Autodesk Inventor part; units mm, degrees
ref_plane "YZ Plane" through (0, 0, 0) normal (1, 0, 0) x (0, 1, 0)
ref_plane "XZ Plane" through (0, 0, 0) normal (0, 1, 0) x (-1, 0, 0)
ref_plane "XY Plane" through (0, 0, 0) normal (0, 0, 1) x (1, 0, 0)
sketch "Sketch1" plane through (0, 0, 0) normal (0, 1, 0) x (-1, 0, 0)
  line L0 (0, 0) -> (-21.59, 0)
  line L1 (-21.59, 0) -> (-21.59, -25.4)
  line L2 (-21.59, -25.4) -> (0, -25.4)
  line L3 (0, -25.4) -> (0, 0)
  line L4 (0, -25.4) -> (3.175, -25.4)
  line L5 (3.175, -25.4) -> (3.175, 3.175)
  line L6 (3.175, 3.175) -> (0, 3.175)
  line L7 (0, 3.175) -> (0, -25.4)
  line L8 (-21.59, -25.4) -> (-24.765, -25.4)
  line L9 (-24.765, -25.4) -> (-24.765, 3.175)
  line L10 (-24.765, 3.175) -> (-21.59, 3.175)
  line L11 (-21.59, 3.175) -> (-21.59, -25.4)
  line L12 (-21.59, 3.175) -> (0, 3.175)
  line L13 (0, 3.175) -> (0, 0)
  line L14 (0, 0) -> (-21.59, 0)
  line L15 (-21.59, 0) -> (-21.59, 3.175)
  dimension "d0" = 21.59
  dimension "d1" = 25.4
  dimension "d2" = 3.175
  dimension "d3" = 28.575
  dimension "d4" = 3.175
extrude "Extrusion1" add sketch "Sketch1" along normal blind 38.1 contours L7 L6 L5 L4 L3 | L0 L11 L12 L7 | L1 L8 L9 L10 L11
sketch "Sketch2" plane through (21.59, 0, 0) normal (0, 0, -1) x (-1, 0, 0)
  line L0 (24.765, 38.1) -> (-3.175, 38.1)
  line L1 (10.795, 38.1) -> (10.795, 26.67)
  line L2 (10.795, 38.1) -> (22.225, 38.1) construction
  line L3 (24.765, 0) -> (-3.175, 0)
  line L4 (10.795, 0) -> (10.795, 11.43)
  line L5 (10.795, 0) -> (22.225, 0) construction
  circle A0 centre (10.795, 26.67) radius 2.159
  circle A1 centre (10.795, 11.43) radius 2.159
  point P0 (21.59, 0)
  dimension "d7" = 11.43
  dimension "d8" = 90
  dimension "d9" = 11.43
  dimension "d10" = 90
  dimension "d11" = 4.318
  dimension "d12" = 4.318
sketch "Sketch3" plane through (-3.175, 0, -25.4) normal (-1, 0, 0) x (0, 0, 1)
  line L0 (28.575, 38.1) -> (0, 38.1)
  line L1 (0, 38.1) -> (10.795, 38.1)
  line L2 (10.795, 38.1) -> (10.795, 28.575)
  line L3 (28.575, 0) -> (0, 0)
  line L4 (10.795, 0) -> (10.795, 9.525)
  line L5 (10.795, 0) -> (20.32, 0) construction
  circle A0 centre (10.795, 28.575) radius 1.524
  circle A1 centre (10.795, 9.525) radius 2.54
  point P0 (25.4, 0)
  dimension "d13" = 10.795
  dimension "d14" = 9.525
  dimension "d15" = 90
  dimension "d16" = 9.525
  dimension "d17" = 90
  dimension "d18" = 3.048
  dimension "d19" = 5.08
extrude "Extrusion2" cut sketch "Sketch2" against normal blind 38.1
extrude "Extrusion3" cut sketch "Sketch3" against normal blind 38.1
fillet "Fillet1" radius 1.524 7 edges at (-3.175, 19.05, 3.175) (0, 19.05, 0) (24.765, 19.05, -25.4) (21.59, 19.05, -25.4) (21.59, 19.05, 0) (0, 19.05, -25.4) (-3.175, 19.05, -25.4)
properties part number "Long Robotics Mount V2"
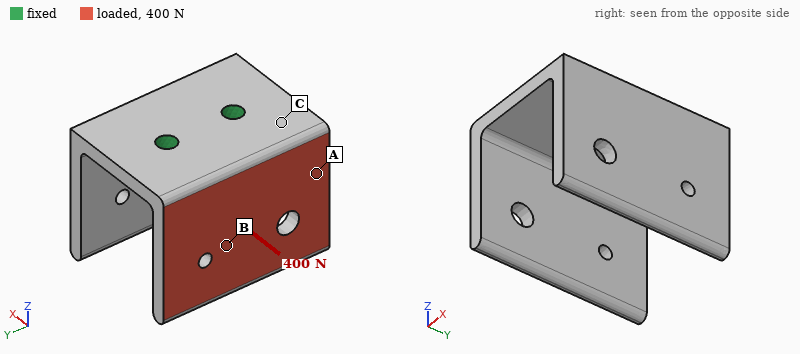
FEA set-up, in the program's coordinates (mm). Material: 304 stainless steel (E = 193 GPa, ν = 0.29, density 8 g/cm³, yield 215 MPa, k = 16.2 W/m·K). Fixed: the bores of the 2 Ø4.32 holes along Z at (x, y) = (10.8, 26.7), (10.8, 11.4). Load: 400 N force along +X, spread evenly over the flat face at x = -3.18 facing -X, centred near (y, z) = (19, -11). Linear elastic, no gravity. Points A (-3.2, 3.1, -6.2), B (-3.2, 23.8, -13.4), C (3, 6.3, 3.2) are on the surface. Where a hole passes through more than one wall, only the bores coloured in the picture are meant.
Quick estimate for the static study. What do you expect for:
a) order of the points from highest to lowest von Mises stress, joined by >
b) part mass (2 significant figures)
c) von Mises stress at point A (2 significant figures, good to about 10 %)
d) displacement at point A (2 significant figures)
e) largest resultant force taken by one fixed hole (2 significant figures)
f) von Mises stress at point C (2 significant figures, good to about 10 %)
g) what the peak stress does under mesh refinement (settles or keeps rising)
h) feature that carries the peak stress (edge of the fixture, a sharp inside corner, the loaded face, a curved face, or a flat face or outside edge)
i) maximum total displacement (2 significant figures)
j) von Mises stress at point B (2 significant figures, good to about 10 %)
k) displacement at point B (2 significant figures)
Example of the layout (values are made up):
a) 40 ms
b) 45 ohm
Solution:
a) C > A > B
b) 74 g
c) 37 MPa
d) 0.034 mm
e) 200 N
f) 65 MPa
g) keeps rising
h) edge of the fixture
i) 0.11 mm
j) 14 MPa
k) 0.060 mm
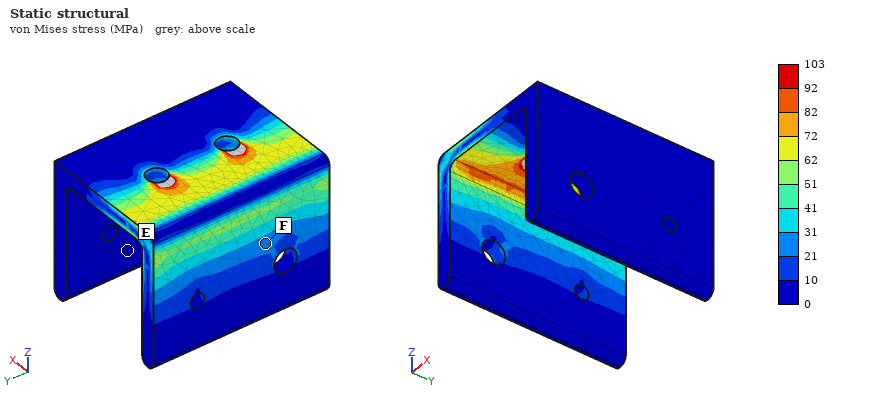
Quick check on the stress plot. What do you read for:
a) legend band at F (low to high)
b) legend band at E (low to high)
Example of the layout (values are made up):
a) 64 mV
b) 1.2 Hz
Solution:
a) 21 to 31 MPa
b) 0 to 10 MPa
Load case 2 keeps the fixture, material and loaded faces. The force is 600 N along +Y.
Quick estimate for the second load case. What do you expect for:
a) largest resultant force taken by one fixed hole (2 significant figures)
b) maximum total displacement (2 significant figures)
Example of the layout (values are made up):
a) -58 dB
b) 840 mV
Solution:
a) 640 N
b) 34 µm
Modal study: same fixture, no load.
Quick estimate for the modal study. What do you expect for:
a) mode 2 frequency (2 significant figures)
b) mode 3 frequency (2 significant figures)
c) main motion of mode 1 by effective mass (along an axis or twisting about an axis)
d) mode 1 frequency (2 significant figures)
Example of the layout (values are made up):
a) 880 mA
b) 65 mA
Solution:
a) 2300 Hz
b) 3900 Hz
c) along X
d) 2200 Hz
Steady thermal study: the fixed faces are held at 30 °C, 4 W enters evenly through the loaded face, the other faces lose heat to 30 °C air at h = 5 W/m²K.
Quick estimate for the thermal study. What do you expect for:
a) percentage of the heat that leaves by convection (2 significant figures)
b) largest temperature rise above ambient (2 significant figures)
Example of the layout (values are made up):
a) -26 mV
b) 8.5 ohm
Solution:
a) 9.3 %
b) 46 K
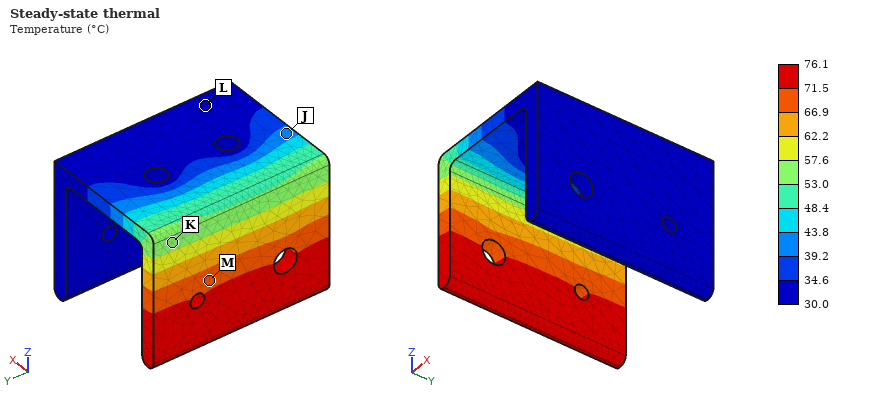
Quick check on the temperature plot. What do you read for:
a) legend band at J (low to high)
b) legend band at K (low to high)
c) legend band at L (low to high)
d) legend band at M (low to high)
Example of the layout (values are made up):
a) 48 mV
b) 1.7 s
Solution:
a) 39.2 to 43.8 °C
b) 53.0 to 57.6 °C
c) 30.0 to 34.6 °C
d) 66.9 to 71.5 °C
